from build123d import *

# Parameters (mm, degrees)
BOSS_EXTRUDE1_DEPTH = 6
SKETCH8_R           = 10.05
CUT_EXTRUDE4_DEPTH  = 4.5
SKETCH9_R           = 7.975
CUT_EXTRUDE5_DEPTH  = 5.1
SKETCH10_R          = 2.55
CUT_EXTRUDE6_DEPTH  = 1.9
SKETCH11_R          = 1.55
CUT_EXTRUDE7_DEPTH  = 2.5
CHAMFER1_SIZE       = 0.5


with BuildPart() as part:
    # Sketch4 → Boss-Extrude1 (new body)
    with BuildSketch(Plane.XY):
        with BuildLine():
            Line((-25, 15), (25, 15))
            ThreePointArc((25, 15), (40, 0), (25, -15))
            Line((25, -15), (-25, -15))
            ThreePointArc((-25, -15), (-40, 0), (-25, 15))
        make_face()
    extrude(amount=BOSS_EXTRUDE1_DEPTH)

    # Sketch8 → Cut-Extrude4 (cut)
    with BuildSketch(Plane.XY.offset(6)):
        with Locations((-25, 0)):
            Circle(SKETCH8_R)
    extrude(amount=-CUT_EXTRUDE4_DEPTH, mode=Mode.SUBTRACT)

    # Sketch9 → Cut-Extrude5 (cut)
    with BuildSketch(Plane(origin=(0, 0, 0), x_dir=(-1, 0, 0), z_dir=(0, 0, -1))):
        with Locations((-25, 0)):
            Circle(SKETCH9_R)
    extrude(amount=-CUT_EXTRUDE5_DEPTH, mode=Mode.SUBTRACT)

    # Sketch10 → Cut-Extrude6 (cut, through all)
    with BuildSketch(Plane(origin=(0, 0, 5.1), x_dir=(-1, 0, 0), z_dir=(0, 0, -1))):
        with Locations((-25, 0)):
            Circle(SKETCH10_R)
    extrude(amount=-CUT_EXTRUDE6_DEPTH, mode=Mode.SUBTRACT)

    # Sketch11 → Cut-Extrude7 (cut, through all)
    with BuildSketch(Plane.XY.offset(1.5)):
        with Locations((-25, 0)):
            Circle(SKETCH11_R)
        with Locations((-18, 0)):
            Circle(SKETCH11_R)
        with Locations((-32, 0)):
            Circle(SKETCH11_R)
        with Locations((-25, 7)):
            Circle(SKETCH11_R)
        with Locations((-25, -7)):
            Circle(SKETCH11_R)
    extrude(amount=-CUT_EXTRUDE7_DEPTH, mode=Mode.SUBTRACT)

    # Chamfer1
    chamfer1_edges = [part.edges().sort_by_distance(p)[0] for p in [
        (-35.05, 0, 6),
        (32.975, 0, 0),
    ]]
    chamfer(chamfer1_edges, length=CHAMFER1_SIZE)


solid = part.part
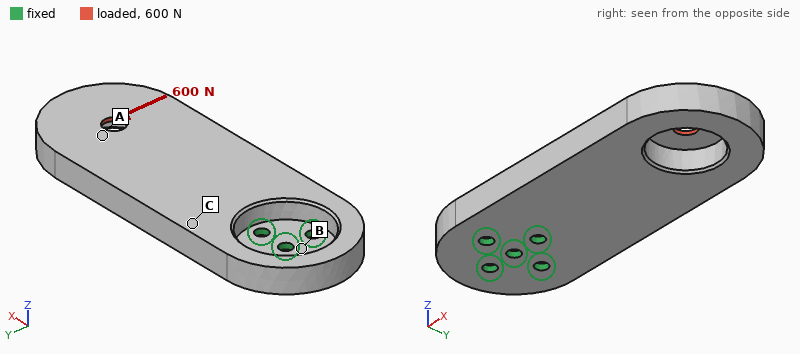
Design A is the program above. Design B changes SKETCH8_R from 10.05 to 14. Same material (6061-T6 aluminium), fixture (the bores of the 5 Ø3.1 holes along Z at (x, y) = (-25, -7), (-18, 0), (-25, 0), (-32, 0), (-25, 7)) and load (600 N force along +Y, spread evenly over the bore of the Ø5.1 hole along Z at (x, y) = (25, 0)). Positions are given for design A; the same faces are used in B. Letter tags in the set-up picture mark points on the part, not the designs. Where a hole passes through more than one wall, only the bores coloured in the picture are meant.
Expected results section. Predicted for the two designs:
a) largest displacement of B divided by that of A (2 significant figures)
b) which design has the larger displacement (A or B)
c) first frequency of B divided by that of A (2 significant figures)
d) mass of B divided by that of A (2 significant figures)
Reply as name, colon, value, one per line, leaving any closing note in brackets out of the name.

largest displacement of B divided by that of A: 1.3
which design has the larger displacement: B
first frequency of B divided by that of A: 0.63
mass of B divided by that of A: 0.87
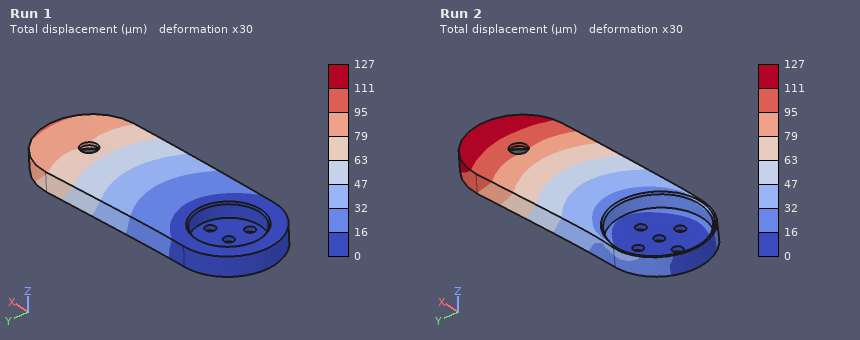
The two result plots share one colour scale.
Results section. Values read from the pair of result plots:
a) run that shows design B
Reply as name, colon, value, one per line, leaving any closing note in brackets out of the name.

run that shows design B: Run 2
